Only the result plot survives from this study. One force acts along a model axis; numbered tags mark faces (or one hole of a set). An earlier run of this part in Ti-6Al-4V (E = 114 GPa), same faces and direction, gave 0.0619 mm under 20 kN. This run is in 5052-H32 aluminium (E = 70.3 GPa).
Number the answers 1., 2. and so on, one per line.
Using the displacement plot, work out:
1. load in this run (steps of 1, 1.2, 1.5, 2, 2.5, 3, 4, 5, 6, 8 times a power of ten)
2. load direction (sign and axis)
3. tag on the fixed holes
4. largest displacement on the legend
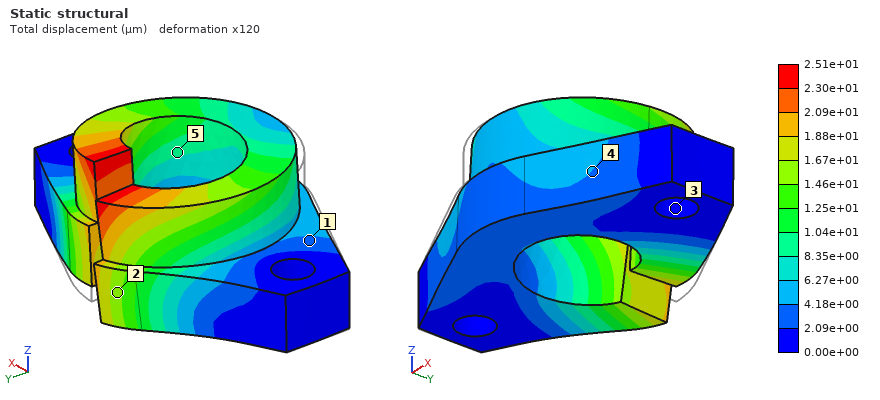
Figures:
1. 5 kN
2. +X
3. 3
4. 2.51e+01 µm
